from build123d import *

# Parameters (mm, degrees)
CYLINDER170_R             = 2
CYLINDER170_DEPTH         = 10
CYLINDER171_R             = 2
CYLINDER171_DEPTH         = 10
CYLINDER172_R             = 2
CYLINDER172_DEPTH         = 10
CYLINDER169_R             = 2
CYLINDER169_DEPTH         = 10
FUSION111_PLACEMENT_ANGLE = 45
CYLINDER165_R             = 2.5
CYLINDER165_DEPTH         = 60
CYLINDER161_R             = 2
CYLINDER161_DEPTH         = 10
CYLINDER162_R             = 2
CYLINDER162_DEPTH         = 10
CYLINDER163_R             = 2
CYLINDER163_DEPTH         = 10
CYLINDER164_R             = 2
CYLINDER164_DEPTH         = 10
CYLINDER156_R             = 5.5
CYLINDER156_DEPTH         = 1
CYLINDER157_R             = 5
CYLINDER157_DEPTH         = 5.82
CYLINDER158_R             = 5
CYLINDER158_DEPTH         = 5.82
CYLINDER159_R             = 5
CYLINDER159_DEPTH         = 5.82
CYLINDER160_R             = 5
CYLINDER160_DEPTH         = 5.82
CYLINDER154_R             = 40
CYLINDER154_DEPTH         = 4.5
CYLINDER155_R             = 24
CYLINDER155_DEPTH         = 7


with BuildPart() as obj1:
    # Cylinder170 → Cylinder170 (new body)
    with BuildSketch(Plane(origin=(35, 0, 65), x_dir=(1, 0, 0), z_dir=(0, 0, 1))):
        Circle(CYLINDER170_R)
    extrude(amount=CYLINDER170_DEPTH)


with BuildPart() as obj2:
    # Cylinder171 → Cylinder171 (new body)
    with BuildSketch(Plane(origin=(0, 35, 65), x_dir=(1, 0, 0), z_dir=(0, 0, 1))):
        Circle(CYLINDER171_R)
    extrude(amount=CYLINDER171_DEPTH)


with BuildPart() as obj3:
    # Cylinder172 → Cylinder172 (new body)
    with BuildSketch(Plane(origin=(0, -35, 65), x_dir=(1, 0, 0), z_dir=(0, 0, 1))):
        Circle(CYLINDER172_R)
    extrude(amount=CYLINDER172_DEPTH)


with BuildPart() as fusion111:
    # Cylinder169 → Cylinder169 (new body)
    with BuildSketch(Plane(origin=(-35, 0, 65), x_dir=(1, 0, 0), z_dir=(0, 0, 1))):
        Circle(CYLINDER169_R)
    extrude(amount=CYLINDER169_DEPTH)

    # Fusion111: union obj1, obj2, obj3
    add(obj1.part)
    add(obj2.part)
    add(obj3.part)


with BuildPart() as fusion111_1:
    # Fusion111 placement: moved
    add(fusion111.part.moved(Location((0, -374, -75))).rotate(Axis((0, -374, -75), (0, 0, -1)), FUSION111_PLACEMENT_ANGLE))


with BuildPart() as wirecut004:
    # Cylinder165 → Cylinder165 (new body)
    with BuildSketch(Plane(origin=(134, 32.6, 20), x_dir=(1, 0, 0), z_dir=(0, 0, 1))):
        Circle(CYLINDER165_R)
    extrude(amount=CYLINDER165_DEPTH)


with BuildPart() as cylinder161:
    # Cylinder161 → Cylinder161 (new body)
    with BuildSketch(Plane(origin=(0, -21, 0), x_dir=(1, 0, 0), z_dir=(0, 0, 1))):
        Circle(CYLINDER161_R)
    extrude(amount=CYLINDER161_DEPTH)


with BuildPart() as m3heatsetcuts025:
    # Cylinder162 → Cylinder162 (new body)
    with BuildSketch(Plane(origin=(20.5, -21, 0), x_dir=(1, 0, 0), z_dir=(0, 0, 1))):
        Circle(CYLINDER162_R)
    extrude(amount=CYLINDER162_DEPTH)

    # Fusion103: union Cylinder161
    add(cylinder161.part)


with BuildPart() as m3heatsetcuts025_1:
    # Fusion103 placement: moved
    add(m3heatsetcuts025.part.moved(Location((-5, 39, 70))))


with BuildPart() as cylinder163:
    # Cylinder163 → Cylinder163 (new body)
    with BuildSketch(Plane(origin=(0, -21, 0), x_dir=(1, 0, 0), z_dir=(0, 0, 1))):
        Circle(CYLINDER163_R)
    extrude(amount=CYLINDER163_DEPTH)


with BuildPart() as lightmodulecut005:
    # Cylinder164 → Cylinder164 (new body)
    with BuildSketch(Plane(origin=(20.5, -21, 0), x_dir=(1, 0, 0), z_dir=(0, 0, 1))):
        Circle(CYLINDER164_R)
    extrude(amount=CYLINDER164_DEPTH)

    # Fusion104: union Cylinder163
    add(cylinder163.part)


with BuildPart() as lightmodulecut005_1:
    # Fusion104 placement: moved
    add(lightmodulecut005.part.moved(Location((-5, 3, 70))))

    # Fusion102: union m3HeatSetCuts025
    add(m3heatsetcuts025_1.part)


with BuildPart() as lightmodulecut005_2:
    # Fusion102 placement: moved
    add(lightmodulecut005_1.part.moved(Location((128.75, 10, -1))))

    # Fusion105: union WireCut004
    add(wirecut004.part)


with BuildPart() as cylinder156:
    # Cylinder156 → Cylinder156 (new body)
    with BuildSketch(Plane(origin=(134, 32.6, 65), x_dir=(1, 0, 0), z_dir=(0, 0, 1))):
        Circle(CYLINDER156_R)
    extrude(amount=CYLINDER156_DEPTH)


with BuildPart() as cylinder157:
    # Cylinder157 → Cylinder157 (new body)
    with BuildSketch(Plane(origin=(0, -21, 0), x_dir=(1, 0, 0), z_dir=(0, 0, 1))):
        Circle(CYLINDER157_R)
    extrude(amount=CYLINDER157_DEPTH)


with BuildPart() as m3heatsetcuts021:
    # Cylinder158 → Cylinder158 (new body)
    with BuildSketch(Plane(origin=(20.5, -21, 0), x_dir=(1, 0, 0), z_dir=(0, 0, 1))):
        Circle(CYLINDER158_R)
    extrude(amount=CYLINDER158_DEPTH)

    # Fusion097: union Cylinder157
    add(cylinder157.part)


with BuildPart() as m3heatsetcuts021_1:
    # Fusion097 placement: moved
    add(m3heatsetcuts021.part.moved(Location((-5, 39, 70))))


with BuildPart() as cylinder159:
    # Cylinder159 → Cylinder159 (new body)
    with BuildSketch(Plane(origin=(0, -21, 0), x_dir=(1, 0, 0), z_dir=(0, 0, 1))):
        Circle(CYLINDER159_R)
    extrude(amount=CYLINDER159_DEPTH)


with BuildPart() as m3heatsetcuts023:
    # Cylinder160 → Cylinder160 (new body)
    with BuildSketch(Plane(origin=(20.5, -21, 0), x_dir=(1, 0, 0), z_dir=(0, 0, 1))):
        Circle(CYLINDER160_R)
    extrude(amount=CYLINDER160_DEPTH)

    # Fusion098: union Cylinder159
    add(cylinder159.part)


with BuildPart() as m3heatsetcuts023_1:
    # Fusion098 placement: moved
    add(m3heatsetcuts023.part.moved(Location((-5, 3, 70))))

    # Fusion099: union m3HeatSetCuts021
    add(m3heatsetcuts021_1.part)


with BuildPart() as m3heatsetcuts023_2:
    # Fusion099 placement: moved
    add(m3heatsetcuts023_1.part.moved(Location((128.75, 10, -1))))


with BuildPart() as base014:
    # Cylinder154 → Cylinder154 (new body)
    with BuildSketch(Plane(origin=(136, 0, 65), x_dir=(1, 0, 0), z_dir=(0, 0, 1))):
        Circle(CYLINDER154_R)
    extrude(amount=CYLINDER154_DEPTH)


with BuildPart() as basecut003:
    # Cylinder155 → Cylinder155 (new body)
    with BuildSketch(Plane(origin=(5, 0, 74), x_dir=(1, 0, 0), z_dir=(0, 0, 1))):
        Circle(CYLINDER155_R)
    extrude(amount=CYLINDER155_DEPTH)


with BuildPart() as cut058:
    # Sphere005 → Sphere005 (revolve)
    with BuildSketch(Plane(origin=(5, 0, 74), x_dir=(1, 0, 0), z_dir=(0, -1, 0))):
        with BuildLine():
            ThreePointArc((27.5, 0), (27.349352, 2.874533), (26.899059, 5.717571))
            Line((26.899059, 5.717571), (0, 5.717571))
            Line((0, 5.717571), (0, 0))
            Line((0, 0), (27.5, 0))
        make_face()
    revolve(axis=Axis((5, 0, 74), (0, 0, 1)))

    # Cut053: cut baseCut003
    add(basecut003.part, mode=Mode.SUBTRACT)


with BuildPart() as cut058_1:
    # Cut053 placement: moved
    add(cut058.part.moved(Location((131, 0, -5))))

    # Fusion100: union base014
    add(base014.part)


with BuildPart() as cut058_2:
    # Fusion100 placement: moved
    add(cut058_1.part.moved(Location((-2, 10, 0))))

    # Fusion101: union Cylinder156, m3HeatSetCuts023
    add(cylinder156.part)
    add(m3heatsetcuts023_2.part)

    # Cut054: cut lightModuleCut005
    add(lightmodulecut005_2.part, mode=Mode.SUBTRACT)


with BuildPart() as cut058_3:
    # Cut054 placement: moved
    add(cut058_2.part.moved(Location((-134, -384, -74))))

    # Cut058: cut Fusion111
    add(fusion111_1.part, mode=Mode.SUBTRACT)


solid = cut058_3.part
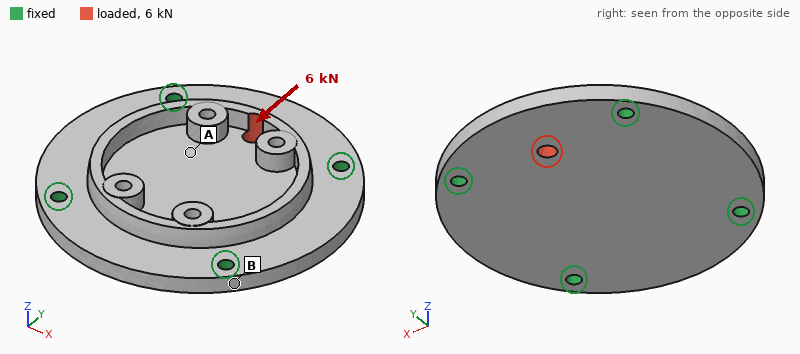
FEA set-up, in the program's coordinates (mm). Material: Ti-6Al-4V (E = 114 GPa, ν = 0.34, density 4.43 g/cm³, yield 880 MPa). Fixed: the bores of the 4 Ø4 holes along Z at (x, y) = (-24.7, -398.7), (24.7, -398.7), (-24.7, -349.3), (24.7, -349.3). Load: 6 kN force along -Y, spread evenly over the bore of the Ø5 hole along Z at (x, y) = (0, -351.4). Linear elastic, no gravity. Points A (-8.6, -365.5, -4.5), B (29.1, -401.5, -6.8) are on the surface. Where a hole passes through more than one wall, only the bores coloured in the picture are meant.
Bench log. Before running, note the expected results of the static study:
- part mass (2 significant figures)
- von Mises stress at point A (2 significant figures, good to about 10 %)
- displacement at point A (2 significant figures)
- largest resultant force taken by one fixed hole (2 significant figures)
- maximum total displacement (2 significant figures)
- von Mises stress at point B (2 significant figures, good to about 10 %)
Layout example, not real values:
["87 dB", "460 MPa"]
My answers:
["120 g", "34 MPa", "6.4 µm", "1.8 kN", "35 µm", "15 MPa"]
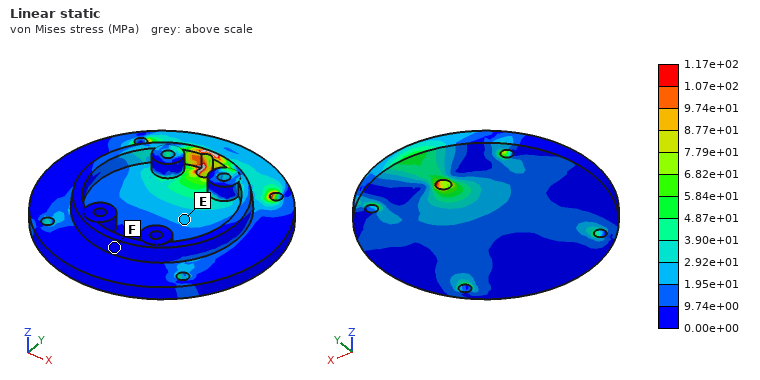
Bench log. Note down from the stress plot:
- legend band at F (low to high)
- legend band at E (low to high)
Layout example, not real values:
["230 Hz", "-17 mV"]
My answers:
["0.00e+00 to 9.74e+00 MPa", "1.95e+01 to 2.92e+01 MPa"]
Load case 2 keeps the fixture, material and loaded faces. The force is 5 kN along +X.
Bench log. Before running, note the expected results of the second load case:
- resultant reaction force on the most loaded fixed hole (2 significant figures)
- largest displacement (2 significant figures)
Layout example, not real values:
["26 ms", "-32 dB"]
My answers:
["2.2 kN", "9.1 µm"]
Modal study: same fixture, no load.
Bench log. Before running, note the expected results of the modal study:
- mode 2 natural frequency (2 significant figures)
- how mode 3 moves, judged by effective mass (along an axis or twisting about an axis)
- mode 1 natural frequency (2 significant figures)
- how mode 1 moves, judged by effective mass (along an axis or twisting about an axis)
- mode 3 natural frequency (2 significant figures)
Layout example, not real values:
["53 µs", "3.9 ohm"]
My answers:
["8000 Hz", "twisting about X", "7200 Hz", "along Z", "8800 Hz"]
